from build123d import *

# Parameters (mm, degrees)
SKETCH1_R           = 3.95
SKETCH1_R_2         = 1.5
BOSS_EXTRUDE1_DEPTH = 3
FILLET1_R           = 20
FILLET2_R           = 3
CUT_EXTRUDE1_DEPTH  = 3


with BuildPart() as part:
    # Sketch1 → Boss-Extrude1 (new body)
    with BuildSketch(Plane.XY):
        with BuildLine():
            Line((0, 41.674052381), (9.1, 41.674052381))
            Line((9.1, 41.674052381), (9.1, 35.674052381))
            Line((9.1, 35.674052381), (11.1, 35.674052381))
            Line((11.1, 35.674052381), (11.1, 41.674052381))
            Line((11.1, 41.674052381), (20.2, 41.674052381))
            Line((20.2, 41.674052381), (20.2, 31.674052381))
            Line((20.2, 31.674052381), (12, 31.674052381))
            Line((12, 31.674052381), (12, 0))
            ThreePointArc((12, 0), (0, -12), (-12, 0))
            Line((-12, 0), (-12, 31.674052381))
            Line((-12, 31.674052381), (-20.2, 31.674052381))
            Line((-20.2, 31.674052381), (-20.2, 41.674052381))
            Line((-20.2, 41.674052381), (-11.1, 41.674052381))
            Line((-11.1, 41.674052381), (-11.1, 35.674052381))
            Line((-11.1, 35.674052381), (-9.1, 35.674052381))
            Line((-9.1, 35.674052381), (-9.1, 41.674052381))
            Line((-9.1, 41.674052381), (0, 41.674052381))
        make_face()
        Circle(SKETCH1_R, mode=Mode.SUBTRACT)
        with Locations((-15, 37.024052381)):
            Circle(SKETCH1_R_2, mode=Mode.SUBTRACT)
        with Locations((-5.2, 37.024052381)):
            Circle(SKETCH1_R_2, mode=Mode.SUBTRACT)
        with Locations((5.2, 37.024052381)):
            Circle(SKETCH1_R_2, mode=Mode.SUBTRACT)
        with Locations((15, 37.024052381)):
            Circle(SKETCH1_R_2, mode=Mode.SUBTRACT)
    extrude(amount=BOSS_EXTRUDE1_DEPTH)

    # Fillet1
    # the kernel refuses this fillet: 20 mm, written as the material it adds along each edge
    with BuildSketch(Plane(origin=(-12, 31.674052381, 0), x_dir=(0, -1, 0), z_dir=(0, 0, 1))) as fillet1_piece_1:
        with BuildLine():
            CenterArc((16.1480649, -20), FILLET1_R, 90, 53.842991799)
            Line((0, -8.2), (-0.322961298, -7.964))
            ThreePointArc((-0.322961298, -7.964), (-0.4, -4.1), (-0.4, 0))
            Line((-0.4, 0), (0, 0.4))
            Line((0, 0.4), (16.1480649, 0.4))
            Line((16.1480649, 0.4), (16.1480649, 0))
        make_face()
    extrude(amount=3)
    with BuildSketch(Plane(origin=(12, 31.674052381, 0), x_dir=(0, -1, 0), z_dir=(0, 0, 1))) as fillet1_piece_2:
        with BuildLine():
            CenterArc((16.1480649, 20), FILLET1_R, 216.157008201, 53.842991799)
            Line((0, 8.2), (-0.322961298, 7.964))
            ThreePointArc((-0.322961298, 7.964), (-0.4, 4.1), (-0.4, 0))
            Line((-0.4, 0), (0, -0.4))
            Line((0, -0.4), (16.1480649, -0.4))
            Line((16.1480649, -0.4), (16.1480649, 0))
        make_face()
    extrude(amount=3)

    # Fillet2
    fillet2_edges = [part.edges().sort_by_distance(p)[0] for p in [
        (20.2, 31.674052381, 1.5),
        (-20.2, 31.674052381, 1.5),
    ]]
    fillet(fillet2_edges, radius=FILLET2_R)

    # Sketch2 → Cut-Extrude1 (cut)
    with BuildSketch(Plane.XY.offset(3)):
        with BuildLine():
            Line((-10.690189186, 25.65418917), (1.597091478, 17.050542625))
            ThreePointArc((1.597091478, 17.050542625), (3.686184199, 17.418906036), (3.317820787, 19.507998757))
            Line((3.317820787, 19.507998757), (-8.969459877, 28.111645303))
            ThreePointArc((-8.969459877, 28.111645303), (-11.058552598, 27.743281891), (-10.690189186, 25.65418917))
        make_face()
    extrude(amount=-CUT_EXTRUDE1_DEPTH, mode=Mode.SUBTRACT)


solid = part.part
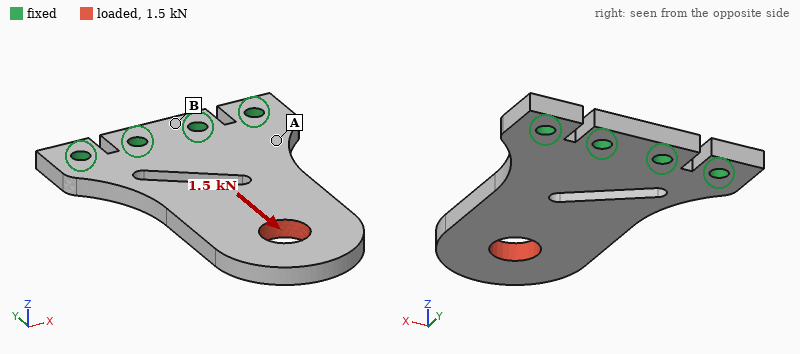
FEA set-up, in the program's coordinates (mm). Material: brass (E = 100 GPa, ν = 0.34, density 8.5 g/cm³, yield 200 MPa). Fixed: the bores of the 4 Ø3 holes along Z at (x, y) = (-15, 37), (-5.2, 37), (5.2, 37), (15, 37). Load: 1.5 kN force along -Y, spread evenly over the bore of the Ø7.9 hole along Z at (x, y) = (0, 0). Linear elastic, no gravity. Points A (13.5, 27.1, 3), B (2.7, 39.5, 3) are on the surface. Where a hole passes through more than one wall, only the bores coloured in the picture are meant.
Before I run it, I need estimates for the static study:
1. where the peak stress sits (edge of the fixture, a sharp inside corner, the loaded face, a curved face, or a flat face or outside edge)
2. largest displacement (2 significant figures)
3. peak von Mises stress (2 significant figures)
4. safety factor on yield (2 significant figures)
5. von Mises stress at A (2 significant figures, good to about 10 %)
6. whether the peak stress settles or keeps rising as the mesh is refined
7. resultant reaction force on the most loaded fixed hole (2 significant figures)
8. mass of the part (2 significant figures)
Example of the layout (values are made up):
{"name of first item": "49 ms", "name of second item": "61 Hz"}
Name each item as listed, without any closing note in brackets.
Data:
{"where the peak stress sits": "a curved face", "largest displacement": "15 µm", "peak von Mises stress": "180 MPa", "safety factor on yield": "1.1", "von Mises stress at A": "24 MPa", "whether the peak stress settles or keeps rising as the mesh is refined": "settles", "resultant reaction force on the most loaded fixed hole": "520 N", "mass of the part": "34 g"}
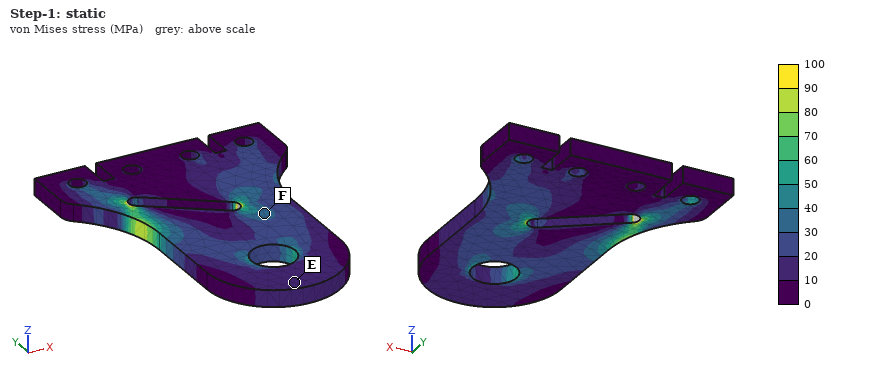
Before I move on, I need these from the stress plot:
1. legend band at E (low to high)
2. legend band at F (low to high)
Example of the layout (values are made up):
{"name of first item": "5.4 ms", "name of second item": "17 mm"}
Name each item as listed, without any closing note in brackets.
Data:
{"legend band at E": "10 to 20 MPa", "legend band at F": "30 to 40 MPa"}
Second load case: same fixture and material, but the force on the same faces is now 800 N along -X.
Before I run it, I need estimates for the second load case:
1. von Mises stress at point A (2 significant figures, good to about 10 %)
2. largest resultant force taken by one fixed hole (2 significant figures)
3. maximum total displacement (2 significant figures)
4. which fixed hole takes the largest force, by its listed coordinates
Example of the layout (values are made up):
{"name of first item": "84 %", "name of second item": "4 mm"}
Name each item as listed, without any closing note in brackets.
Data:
{"von Mises stress at point A": "45 MPa", "largest resultant force taken by one fixed hole": "940 N", "maximum total displacement": "50 µm", "which fixed hole takes the largest force, by its listed coordinates": "(-15, 37)"}
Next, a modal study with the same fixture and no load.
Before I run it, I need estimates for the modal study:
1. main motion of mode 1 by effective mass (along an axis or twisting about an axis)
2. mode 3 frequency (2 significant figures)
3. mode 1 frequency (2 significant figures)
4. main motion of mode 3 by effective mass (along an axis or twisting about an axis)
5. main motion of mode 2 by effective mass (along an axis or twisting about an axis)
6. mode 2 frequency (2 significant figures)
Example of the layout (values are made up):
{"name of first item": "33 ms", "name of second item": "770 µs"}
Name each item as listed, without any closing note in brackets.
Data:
{"main motion of mode 1 by effective mass": "along Z", "mode 3 frequency": "4700 Hz", "mode 1 frequency": "810 Hz", "main motion of mode 3 by effective mass": "along Z", "main motion of mode 2 by effective mass": "twisting about Y", "mode 2 frequency": "3400 Hz"}
